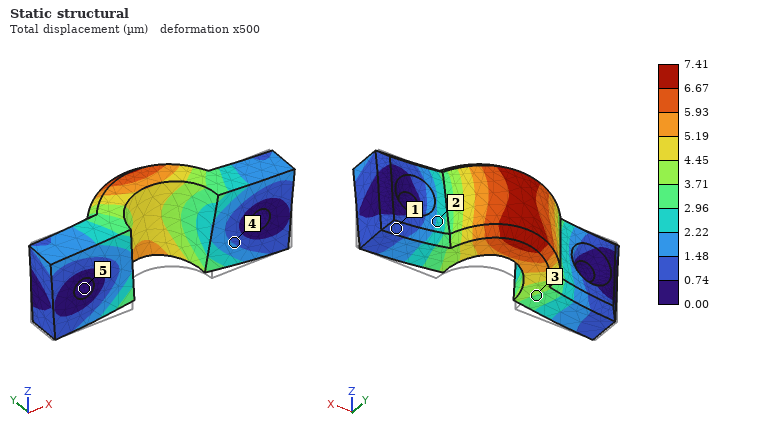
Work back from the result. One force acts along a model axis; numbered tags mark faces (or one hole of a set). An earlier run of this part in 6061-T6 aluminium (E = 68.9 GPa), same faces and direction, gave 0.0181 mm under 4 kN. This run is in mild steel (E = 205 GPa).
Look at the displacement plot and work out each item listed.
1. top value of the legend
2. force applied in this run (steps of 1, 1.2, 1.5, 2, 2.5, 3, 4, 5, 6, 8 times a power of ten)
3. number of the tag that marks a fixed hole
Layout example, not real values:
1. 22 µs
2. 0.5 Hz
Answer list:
1. 7.41 µm
2. 5 kN
3. 5
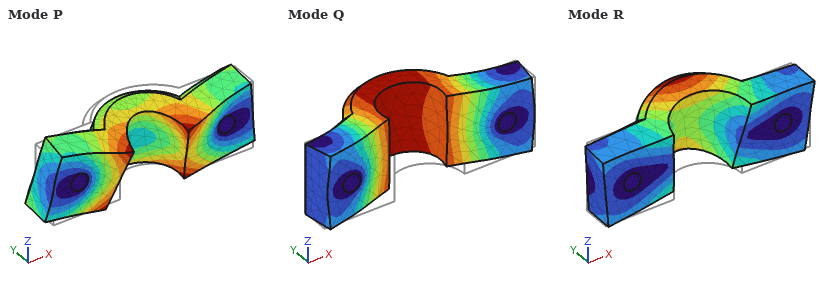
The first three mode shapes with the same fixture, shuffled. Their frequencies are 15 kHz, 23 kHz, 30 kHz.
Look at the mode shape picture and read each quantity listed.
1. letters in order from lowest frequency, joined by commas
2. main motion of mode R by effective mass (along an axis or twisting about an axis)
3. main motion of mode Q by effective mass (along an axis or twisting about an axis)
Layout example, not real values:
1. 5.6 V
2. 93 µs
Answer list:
1. R, Q, P
2. along Z
3. along Y
